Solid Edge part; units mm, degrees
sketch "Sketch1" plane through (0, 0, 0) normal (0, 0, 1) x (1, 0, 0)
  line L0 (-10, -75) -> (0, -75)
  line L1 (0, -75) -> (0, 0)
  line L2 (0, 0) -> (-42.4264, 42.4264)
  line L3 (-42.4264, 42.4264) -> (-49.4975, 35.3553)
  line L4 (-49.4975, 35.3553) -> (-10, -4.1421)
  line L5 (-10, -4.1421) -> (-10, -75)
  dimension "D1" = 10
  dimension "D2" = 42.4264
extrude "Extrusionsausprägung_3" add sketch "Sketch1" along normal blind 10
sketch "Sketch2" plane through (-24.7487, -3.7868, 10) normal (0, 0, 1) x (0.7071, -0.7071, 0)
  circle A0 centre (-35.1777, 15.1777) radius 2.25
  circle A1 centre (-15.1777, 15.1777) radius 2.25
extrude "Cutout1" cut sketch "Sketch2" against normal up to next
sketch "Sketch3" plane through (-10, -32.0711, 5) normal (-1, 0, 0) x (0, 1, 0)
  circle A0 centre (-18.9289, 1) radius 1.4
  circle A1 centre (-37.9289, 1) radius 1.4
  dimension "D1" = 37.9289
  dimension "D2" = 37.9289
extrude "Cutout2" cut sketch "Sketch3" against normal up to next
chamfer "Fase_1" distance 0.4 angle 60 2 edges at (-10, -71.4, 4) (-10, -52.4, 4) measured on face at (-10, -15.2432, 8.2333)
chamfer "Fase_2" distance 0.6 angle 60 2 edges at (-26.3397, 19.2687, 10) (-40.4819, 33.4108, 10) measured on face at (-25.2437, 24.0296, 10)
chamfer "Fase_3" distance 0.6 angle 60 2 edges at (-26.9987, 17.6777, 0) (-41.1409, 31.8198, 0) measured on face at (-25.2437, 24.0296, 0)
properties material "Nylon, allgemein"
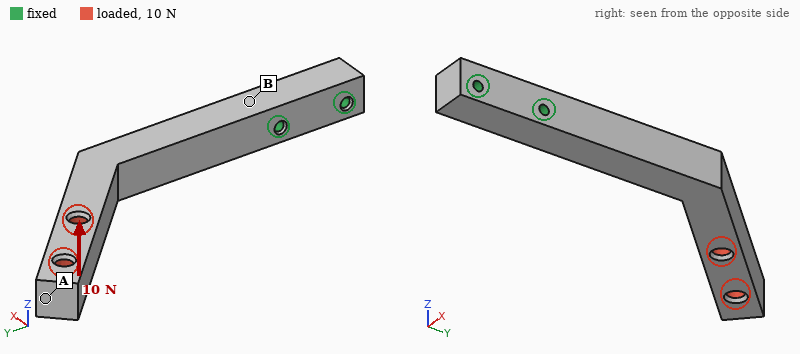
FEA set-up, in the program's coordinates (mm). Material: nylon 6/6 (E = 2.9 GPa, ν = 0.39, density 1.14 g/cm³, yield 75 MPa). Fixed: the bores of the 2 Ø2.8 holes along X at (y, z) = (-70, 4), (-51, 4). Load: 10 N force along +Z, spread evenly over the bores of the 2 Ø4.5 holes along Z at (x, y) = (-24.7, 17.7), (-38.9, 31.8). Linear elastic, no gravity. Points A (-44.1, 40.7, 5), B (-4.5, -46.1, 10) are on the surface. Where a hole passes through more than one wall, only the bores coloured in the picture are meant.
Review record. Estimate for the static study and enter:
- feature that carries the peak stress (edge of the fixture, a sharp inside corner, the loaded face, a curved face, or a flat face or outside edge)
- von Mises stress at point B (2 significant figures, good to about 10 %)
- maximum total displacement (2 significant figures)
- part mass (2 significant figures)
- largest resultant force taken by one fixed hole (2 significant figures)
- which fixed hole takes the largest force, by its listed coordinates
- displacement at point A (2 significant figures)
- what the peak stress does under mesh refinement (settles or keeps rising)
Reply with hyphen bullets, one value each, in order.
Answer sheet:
- edge of the fixture
- 4.7 MPa
- 1.3 mm
- 14 g
- 40 N
- (-51, 4)
- 1.3 mm
- keeps rising
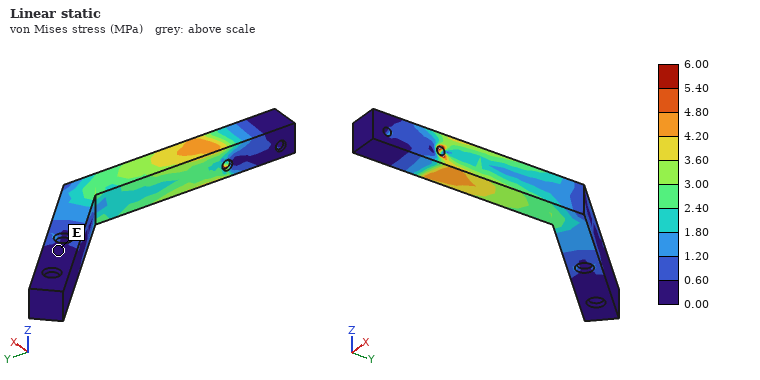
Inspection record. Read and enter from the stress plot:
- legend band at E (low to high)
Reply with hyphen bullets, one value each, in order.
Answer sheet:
- 0.00 to 0.60 MPa
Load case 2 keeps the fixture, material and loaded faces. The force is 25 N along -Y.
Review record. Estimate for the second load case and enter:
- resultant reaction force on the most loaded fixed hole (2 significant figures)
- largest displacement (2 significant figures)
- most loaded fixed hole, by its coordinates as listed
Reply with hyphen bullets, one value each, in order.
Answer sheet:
- 23 N
- 1.3 mm
- (-51, 4)
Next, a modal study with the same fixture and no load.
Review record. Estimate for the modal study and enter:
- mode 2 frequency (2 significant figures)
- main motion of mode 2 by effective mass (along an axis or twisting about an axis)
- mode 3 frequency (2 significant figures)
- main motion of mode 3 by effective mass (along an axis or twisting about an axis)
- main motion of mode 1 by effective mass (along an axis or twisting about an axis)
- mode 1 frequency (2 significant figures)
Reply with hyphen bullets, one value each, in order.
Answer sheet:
- 250 Hz
- along X
- 940 Hz
- along Z
- along Z
- 230 Hz
